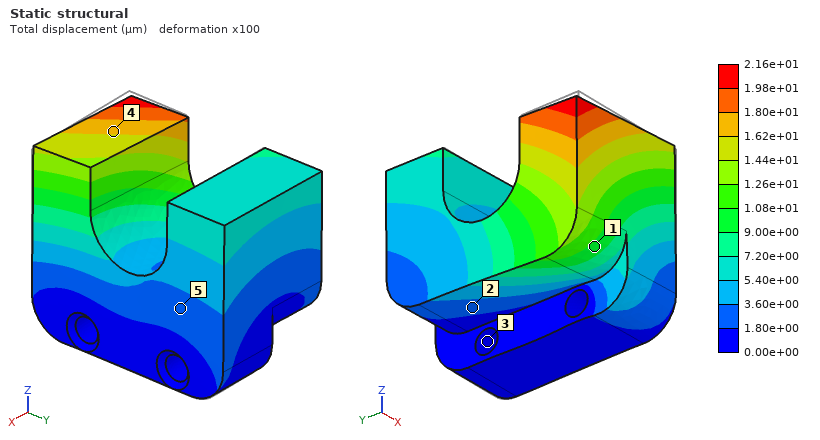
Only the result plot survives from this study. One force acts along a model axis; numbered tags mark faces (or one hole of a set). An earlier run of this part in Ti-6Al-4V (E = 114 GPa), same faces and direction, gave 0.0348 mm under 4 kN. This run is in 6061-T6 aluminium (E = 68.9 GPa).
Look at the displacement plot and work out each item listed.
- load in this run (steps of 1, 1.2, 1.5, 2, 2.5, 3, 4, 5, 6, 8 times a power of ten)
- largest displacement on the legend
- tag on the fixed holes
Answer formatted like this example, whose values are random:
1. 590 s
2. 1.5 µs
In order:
1. 1.5 kN
2. 2.16e+01 µm
3. 3
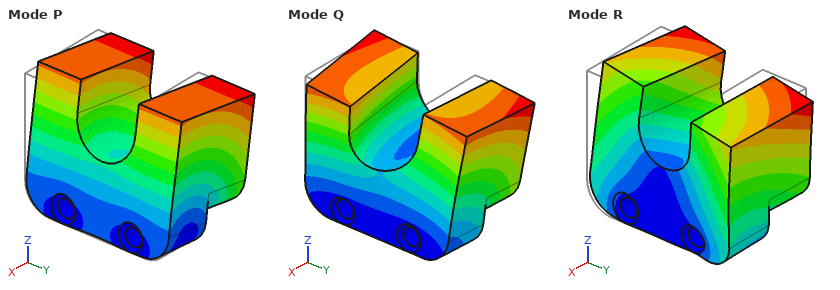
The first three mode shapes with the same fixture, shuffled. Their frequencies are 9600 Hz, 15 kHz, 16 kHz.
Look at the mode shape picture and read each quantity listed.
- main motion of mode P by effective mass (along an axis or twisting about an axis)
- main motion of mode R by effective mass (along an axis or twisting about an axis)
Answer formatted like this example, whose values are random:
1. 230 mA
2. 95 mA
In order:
1. along X
2. along Y
